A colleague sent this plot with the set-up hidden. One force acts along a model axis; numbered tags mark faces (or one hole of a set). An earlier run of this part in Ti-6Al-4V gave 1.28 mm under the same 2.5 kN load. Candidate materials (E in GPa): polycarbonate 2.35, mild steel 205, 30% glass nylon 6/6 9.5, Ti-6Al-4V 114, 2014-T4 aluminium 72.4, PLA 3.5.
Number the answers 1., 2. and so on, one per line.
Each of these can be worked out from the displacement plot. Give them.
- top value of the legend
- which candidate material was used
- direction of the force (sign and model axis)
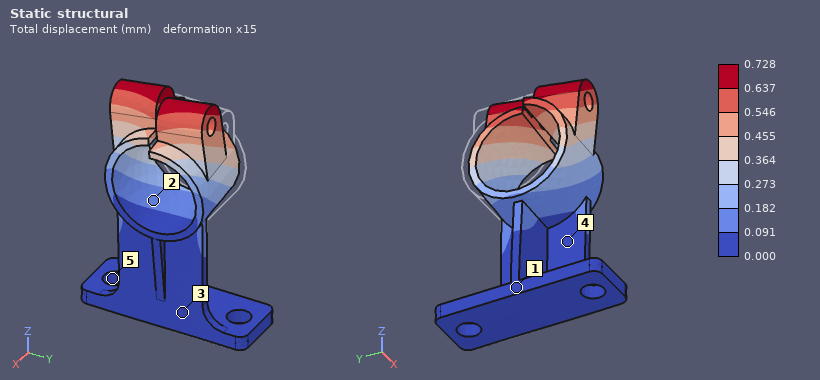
1. 0.728 mm
2. mild steel
3. -Y
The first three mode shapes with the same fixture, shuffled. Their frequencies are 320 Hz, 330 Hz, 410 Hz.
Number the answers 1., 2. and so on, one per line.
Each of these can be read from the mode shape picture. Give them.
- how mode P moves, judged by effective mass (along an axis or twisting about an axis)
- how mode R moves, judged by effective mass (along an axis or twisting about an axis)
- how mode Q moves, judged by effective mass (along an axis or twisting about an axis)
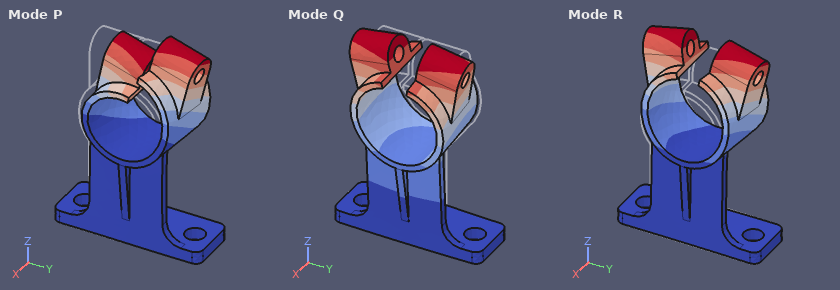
1. along Y
2. along X
3. along X
